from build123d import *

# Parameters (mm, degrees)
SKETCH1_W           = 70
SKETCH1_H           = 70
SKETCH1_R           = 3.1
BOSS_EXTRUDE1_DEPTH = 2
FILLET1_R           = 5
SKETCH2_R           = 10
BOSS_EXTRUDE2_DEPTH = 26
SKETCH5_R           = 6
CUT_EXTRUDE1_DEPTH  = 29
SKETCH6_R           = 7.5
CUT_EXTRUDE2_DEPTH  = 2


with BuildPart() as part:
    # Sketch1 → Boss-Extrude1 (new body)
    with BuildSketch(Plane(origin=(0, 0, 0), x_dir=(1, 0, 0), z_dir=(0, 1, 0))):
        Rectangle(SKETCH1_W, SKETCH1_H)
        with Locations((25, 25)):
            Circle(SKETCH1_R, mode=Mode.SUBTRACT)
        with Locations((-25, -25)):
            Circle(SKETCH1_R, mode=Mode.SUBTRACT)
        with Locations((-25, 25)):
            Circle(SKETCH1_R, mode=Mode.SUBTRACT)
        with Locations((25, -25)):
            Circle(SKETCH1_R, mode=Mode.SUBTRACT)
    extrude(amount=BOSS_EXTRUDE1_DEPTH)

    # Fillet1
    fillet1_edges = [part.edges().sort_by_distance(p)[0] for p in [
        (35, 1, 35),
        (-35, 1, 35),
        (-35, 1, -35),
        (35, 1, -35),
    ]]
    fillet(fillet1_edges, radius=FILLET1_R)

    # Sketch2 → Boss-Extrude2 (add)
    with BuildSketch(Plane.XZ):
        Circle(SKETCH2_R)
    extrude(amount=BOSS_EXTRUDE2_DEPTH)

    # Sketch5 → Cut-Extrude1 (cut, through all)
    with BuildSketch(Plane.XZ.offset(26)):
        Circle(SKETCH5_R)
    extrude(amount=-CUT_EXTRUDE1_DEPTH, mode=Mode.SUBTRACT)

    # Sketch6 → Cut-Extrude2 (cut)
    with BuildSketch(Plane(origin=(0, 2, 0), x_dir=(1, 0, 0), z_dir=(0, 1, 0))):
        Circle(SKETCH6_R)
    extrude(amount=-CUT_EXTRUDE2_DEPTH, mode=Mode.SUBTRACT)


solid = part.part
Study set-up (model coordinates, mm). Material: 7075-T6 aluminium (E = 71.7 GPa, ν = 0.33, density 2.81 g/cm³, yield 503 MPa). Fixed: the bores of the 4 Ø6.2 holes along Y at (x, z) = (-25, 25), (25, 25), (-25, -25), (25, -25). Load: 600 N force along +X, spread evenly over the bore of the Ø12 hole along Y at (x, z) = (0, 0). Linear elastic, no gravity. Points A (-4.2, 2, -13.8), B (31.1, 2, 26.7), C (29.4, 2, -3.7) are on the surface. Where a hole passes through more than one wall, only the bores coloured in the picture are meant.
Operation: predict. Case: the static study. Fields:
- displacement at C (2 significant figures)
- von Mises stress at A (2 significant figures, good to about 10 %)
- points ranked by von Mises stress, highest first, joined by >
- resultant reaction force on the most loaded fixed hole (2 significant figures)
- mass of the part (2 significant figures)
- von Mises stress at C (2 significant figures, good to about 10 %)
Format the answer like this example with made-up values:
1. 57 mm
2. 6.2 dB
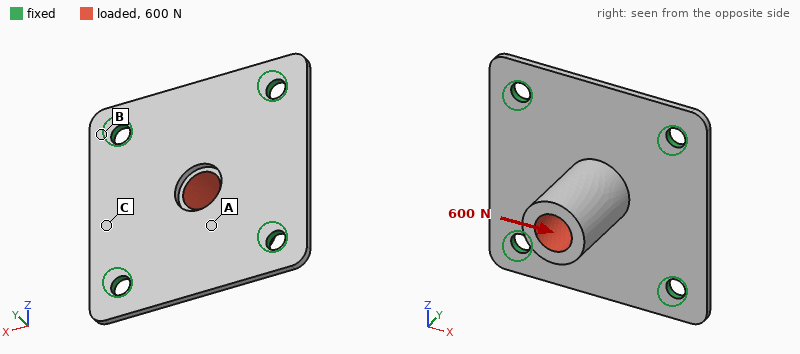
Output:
1. 0.043 mm
2. 47 MPa
3. A > C > B
4. 200 N
5. 40 g
6. 26 MPa
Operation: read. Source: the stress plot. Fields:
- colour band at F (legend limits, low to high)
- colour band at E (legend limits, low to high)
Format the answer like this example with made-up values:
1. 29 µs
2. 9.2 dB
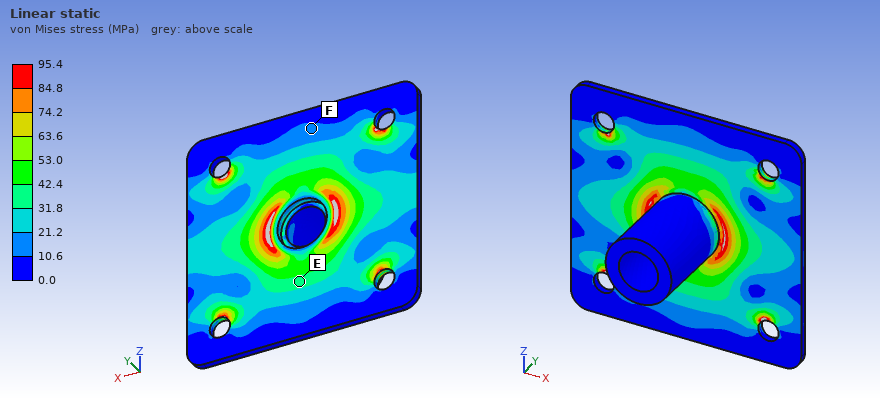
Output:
1. 10.6 to 21.2 MPa
2. 31.8 to 42.4 MPa
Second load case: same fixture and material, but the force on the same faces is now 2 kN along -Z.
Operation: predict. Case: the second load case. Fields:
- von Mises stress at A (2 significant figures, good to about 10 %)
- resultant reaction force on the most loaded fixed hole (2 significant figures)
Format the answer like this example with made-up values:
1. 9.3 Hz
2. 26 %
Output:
1. 210 MPa
2. 660 N
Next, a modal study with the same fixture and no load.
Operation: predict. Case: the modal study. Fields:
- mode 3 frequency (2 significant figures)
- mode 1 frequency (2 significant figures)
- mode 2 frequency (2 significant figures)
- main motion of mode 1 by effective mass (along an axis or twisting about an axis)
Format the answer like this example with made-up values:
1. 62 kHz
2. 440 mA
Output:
1. 2400 Hz
2. 2200 Hz
3. 2400 Hz
4. along Y
